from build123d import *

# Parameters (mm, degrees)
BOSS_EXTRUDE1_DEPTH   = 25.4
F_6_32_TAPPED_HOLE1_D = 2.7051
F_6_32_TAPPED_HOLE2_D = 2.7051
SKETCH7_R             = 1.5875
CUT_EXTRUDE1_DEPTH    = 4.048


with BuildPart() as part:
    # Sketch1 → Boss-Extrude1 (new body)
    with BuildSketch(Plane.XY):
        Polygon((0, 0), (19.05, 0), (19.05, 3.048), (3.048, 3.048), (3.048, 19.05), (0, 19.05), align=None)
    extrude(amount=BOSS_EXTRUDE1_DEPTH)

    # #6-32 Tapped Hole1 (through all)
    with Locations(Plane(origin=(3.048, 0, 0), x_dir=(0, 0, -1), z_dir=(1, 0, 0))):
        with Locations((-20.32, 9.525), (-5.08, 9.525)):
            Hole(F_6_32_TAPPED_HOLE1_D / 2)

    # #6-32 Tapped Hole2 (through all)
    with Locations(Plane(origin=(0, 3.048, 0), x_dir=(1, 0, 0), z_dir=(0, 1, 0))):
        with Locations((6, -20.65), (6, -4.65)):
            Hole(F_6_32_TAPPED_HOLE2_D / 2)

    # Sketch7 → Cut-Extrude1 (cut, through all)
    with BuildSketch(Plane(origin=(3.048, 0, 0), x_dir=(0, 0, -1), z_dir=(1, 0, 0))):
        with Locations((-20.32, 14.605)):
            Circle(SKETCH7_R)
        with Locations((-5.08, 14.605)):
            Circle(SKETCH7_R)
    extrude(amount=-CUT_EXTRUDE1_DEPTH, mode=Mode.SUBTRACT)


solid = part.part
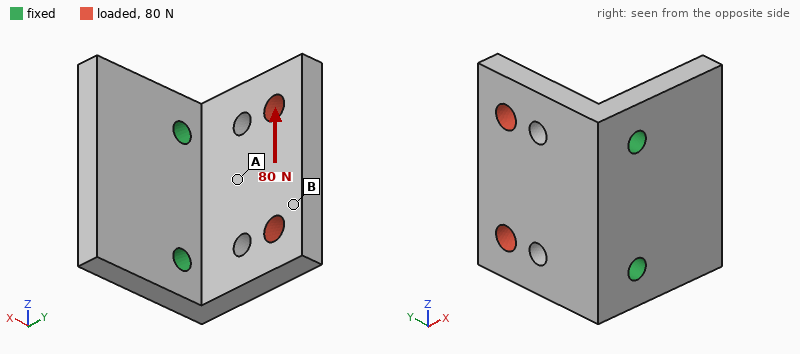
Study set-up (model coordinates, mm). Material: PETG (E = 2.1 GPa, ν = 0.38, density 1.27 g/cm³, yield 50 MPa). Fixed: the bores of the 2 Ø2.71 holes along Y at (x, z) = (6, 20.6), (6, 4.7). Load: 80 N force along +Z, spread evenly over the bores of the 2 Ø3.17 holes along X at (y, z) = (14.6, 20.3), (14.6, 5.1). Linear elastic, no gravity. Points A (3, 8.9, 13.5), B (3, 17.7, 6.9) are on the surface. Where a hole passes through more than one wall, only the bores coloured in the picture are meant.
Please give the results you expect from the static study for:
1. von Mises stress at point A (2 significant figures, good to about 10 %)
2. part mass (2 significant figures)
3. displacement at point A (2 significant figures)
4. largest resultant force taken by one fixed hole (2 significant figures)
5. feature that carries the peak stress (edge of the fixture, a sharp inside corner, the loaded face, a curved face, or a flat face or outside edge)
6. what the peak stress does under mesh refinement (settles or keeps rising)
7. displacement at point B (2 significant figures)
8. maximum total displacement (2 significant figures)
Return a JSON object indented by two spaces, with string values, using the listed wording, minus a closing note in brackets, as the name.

{
  "von Mises stress at point A": "4.0 MPa",
  "part mass": "3.3 g",
  "displacement at point A": "0.048 mm",
  "largest resultant force taken by one fixed hole": "73 N",
  "feature that carries the peak stress": "edge of the fixture",
  "what the peak stress does under mesh refinement": "keeps rising",
  "displacement at point B": "0.11 mm",
  "maximum total displacement": "0.13 mm"
}
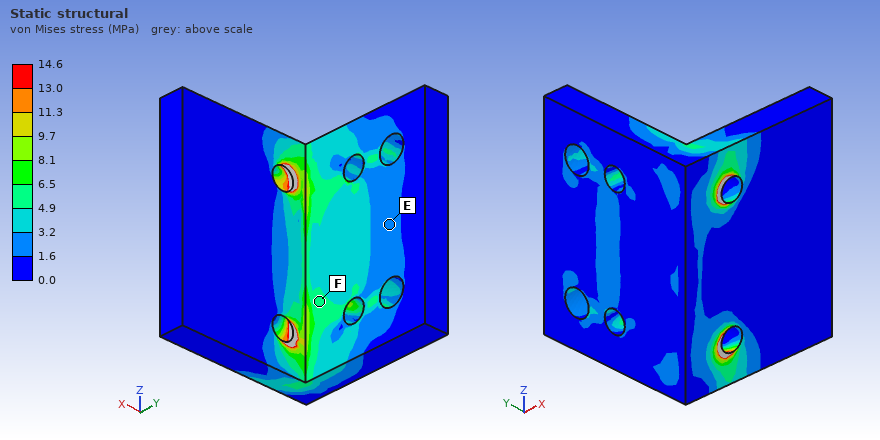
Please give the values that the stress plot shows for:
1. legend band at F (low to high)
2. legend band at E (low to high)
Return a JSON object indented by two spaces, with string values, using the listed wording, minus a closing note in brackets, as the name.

{
  "legend band at F": "4.9 to 6.5 MPa",
  "legend band at E": "1.6 to 3.2 MPa"
}
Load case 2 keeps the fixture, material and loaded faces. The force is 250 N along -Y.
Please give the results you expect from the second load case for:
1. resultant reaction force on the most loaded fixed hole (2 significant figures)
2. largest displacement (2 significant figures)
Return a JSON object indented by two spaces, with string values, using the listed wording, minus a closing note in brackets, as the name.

{
  "resultant reaction force on the most loaded fixed hole": "130 N",
  "largest displacement": "0.40 mm"
}
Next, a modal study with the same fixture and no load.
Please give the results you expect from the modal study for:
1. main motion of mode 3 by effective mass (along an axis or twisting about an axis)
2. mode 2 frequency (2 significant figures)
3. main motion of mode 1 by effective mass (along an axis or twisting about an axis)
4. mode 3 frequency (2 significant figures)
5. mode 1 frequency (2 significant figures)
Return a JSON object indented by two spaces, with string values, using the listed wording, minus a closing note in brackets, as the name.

{
  "main motion of mode 3 by effective mass": "along Y",
  "mode 2 frequency": "3100 Hz",
  "main motion of mode 1 by effective mass": "along X",
  "mode 3 frequency": "3600 Hz",
  "mode 1 frequency": "1600 Hz"
}
